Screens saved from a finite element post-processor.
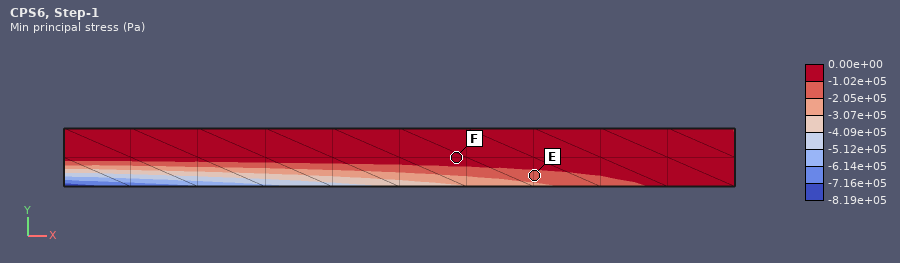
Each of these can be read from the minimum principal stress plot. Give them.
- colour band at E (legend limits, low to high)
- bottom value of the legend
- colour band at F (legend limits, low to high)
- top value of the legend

-2.05e+05 to -1.02e+05 Pa
-8.19e+05 Pa
-1.02e+05 to 0.00e+00 Pa
0.00e+00 Pa
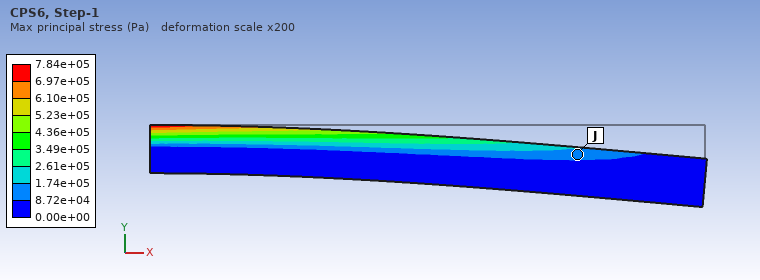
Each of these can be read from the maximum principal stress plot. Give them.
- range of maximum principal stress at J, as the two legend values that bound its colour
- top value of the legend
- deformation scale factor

8.72e+04 to 1.74e+05 Pa
7.84e+05 Pa
200
